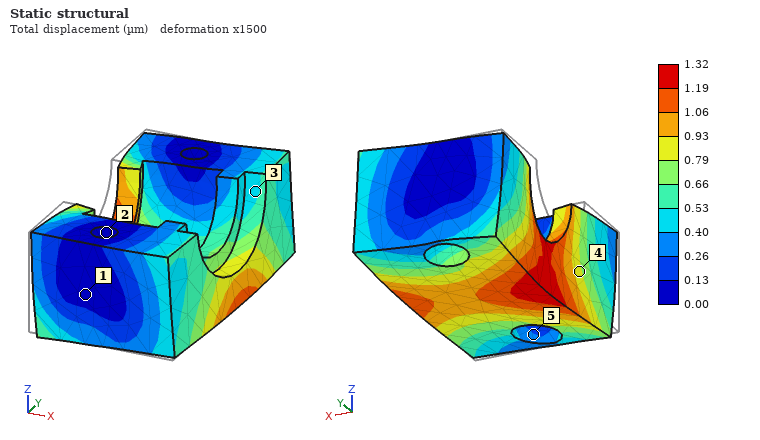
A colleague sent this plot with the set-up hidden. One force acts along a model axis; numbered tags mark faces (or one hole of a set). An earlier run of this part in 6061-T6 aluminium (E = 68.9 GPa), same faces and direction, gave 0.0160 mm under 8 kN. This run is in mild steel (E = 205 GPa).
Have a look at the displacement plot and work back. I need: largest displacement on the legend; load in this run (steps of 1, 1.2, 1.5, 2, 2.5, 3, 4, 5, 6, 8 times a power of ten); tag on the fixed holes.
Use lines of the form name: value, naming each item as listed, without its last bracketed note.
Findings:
largest displacement on the legend: 1.32 µm
load in this run: 2 kN
tag on the fixed holes: 2
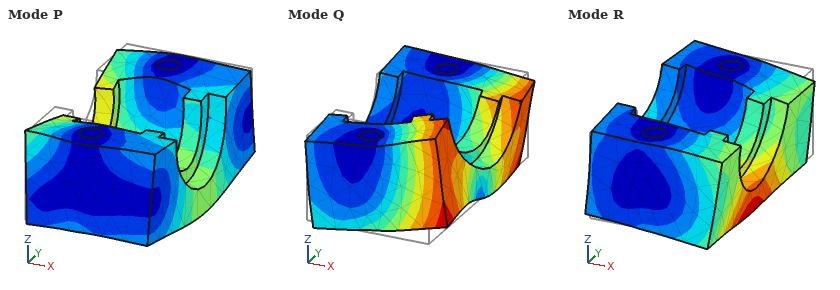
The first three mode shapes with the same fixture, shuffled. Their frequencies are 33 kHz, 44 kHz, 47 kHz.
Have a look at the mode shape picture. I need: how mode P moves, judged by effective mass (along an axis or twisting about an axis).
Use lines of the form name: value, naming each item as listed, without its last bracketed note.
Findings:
how mode P moves, judged by effective mass: along Z
